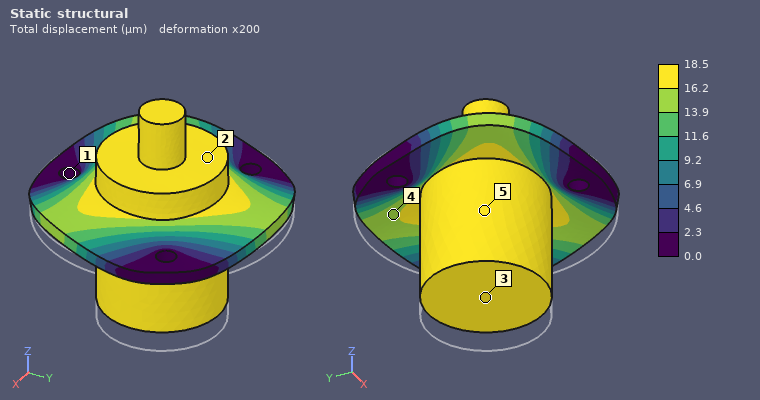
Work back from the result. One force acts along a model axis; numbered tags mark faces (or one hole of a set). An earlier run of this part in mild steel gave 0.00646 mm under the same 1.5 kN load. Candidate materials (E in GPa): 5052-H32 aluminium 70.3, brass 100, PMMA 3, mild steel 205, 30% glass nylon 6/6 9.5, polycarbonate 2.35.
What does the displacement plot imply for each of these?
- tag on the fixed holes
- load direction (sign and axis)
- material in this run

1
+Z
5052-H32 aluminium
